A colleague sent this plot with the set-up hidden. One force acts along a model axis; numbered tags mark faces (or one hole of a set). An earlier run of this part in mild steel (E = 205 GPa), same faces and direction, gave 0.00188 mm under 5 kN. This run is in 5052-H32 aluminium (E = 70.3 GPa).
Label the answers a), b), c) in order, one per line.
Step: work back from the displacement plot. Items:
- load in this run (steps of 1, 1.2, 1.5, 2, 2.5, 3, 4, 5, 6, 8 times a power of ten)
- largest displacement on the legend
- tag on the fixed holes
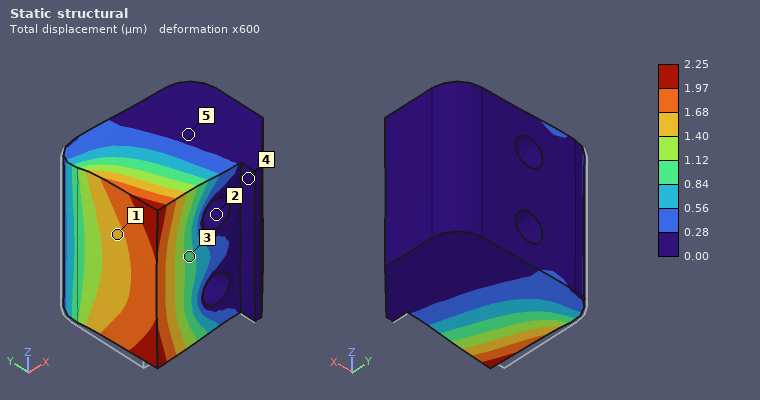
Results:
a) 2 kN
b) 2.25 µm
c) 2
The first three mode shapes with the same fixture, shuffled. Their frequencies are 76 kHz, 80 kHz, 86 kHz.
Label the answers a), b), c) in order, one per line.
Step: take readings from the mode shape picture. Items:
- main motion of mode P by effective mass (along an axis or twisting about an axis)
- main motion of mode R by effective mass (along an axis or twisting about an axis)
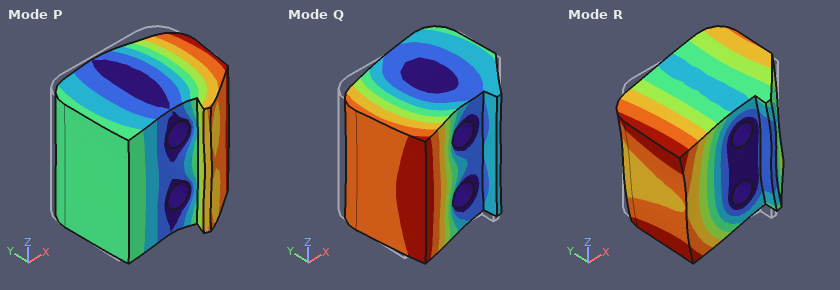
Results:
a) along Y
b) twisting about Y
